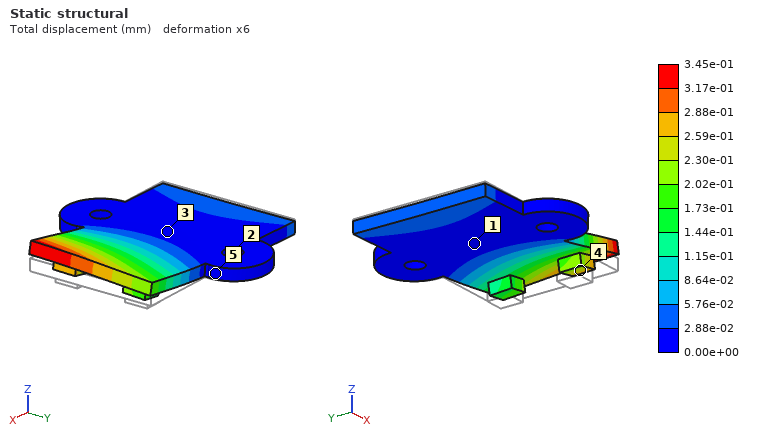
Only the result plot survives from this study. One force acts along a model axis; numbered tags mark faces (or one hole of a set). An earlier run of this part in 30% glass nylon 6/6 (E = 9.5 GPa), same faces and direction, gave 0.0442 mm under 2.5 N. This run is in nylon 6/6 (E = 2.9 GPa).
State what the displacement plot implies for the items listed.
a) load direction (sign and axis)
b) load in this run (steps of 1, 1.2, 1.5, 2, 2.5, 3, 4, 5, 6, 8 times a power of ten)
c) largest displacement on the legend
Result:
+Z
6 N
3.45e-01 mm
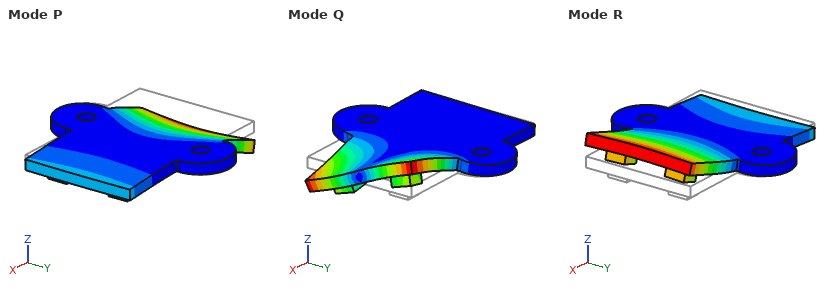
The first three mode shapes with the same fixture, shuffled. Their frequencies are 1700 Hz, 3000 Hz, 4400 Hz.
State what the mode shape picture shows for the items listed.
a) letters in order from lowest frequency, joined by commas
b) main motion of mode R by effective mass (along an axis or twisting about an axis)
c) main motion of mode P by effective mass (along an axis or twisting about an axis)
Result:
R, P, Q
along Z
along Z
